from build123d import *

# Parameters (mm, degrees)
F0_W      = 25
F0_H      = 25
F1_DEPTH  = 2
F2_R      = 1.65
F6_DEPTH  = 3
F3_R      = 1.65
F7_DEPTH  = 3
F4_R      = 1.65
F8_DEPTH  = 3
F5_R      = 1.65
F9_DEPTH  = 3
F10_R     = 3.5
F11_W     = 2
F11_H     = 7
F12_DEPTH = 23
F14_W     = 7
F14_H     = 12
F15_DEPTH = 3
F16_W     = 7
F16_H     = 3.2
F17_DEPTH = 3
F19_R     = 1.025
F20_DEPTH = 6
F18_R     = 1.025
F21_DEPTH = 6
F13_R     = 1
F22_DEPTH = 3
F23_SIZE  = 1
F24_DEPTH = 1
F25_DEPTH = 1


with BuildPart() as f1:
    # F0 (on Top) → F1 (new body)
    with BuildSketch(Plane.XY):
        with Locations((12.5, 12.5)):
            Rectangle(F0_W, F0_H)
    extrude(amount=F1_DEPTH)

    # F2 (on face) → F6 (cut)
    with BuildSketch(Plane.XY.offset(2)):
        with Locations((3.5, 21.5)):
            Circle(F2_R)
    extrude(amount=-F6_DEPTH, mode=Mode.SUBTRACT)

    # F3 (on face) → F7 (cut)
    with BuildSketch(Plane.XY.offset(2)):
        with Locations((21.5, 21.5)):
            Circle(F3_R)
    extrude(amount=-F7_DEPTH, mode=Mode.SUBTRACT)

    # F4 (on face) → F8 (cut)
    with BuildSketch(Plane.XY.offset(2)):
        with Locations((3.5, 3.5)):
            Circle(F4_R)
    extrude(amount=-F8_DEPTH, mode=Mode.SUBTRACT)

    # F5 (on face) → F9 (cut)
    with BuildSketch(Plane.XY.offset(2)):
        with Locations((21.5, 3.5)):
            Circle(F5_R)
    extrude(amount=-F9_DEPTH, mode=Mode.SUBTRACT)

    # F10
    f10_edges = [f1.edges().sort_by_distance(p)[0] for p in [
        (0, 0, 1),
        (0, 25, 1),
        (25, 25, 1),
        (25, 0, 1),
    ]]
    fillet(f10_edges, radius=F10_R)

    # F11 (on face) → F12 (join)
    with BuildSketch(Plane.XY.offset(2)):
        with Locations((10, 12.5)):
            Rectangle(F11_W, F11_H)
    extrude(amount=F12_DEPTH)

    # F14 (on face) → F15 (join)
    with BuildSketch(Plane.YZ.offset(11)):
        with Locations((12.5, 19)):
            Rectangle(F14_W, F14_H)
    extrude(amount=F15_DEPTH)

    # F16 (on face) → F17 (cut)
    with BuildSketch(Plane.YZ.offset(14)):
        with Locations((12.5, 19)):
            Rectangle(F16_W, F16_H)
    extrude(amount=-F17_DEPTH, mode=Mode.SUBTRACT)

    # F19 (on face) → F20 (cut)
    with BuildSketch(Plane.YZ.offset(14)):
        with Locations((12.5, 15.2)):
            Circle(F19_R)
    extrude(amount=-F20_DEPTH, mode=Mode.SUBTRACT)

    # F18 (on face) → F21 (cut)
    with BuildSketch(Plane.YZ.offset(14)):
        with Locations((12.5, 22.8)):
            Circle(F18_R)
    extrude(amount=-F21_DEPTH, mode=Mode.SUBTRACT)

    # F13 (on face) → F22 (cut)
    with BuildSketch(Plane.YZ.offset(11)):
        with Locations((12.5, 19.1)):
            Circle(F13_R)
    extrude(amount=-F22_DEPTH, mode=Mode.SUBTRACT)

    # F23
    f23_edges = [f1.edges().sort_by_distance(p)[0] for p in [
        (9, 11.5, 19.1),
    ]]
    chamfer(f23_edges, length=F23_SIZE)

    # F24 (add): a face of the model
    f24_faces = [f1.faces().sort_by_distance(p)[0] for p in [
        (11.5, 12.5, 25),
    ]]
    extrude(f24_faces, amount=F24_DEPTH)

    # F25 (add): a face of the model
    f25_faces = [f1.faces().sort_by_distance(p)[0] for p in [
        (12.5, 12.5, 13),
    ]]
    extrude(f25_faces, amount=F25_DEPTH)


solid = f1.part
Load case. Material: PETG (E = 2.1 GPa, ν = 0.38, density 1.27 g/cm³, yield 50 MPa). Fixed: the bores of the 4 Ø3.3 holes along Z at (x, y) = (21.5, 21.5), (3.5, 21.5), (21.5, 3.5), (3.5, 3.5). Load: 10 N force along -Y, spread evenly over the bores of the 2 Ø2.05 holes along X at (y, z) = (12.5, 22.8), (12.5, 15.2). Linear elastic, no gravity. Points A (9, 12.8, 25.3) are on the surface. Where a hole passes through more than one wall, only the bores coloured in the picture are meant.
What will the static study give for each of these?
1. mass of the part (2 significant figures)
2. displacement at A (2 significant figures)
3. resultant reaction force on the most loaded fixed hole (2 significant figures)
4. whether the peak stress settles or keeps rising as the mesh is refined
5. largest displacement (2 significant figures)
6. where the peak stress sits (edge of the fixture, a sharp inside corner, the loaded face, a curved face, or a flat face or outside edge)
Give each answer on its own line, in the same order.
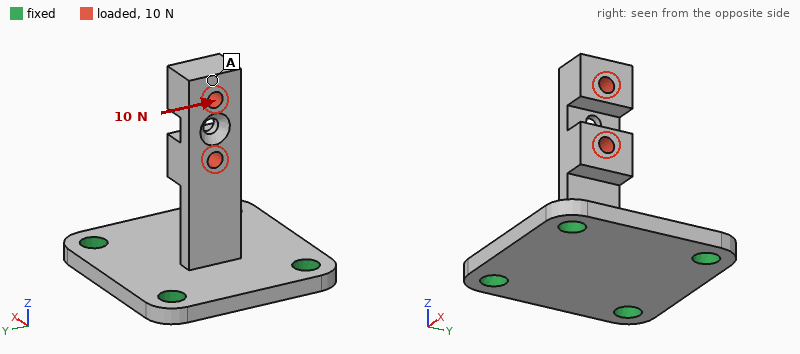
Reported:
2.1 g
0.40 mm
10 N
keeps rising
0.48 mm
a sharp inside corner
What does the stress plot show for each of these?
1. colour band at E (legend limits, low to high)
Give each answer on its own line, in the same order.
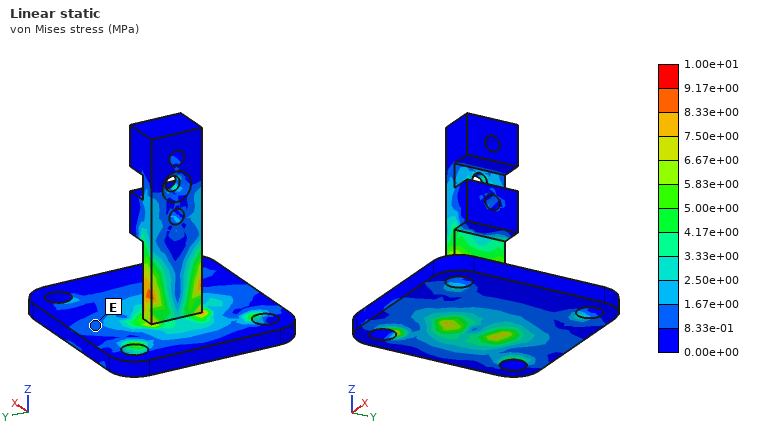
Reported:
8.33e-01 to 1.67e+00 MPa
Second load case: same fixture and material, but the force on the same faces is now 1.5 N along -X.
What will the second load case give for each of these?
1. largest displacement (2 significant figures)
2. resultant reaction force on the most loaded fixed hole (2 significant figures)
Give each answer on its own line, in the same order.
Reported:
0.46 mm
1.0 N
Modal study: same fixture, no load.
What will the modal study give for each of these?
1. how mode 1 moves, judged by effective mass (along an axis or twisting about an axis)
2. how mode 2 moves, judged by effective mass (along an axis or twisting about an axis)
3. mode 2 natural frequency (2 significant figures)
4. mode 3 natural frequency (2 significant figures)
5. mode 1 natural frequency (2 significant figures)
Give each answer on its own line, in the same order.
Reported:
along X
along Y
1200 Hz
2900 Hz
480 Hz
